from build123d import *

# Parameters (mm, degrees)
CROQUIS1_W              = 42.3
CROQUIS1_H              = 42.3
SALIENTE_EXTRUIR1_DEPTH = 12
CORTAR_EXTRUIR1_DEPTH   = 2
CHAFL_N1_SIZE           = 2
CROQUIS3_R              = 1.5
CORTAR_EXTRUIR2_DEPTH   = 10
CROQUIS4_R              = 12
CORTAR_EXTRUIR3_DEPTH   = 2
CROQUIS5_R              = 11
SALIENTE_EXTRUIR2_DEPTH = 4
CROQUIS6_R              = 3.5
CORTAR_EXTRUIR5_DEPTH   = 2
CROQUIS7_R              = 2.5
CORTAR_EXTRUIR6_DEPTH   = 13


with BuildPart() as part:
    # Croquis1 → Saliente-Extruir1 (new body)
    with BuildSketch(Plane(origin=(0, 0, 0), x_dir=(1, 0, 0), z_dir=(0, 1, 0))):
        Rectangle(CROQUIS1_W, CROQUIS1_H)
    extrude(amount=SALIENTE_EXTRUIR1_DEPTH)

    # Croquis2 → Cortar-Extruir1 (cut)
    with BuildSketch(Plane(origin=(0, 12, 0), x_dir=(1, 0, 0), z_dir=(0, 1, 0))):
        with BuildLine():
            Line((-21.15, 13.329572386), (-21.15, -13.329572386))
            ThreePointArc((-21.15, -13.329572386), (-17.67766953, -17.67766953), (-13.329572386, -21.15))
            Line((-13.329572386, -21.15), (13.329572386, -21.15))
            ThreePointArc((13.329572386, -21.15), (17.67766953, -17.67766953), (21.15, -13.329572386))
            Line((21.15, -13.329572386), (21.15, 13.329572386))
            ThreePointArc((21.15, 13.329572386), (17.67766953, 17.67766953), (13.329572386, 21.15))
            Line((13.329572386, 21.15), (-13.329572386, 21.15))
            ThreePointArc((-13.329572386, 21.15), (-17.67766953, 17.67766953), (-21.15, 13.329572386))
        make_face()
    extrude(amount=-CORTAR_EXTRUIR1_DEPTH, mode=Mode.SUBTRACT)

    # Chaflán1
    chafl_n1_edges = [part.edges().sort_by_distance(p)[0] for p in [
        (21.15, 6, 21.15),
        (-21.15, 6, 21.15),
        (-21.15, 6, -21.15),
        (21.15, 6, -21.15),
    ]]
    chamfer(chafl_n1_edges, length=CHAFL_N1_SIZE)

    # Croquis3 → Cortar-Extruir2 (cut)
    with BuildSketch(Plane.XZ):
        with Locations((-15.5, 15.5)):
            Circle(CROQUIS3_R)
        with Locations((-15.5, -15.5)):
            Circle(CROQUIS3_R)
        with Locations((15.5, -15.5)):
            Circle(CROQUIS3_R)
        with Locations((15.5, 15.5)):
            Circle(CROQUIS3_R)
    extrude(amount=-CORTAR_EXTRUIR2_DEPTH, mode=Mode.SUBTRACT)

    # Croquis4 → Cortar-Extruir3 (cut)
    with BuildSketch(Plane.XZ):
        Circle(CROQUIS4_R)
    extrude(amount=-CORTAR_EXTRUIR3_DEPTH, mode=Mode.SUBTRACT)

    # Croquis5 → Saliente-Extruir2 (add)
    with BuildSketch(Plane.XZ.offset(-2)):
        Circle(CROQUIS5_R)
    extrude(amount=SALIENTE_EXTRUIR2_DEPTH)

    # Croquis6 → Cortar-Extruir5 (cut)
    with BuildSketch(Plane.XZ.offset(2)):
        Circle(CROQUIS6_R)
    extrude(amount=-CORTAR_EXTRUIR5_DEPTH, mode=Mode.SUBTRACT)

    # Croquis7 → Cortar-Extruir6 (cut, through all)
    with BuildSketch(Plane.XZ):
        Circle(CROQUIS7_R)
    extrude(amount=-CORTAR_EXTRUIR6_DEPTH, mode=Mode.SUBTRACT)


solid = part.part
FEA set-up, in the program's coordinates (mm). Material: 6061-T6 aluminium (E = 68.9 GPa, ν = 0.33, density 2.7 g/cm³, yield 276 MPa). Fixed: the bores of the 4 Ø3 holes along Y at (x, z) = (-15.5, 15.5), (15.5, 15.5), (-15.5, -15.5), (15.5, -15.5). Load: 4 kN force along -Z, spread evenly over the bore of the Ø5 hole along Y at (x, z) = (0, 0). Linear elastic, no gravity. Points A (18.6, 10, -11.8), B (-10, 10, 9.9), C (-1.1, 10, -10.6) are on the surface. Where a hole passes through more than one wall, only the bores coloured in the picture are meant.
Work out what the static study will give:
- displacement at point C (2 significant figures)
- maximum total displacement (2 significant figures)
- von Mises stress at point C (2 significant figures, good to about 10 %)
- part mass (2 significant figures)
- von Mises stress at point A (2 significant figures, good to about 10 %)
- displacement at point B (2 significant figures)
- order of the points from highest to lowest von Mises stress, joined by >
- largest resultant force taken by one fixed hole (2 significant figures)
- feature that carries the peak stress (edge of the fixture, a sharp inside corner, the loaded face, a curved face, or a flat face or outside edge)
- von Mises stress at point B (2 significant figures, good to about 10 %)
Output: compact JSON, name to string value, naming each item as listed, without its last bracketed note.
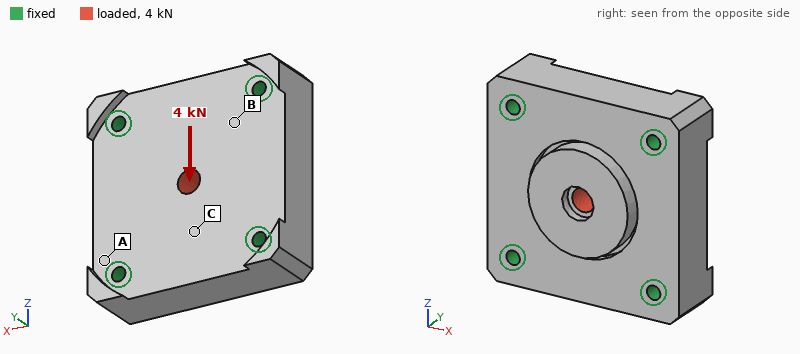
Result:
{"displacement at point C": "3.2 µm", "maximum total displacement": "4.9 µm", "von Mises stress at point C": "6.2 MPa", "part mass": "49 g", "von Mises stress at point A": "3.8 MPa", "displacement at point B": "1.7 µm", "order of the points from highest to lowest von Mises stress, joined by >": "B > C > A", "largest resultant force taken by one fixed hole": "1.1 kN", "feature that carries the peak stress": "a sharp inside corner", "von Mises stress at point B": "12 MPa"}
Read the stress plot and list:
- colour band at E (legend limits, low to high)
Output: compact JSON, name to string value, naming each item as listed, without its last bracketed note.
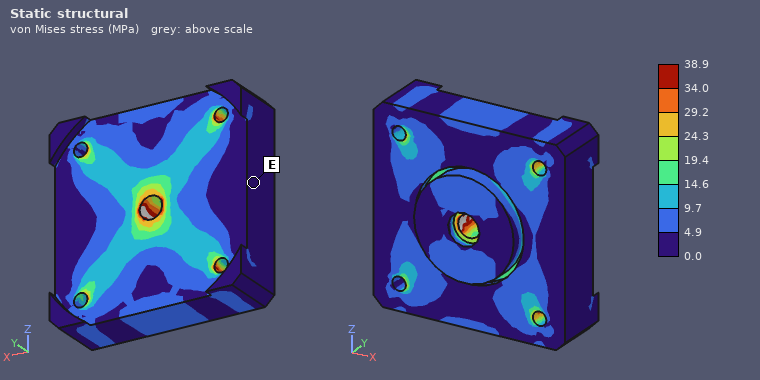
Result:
{"colour band at E": "0.0 to 4.9 MPa"}
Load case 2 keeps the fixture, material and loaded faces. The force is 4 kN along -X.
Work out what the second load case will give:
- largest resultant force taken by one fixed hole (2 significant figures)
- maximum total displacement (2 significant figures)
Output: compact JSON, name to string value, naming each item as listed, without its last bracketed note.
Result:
{"largest resultant force taken by one fixed hole": "1.1 kN", "maximum total displacement": "4.9 µm"}
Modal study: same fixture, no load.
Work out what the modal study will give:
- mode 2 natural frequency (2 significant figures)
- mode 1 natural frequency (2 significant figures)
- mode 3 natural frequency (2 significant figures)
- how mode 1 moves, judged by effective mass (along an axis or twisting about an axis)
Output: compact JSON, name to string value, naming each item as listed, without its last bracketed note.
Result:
{"mode 2 natural frequency": "34 kHz", "mode 1 natural frequency": "24 kHz", "mode 3 natural frequency": "34 kHz", "how mode 1 moves, judged by effective mass": "along Y"}
